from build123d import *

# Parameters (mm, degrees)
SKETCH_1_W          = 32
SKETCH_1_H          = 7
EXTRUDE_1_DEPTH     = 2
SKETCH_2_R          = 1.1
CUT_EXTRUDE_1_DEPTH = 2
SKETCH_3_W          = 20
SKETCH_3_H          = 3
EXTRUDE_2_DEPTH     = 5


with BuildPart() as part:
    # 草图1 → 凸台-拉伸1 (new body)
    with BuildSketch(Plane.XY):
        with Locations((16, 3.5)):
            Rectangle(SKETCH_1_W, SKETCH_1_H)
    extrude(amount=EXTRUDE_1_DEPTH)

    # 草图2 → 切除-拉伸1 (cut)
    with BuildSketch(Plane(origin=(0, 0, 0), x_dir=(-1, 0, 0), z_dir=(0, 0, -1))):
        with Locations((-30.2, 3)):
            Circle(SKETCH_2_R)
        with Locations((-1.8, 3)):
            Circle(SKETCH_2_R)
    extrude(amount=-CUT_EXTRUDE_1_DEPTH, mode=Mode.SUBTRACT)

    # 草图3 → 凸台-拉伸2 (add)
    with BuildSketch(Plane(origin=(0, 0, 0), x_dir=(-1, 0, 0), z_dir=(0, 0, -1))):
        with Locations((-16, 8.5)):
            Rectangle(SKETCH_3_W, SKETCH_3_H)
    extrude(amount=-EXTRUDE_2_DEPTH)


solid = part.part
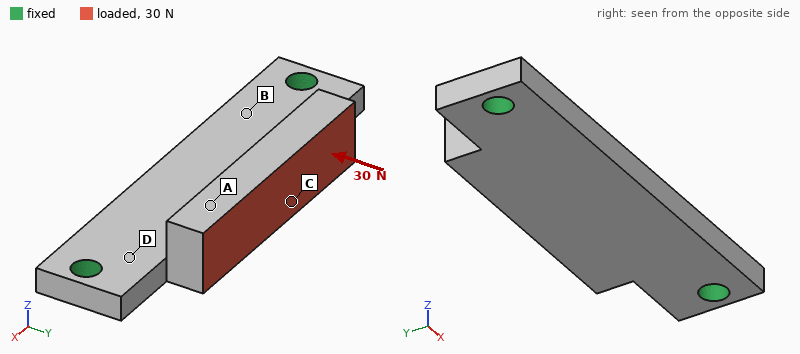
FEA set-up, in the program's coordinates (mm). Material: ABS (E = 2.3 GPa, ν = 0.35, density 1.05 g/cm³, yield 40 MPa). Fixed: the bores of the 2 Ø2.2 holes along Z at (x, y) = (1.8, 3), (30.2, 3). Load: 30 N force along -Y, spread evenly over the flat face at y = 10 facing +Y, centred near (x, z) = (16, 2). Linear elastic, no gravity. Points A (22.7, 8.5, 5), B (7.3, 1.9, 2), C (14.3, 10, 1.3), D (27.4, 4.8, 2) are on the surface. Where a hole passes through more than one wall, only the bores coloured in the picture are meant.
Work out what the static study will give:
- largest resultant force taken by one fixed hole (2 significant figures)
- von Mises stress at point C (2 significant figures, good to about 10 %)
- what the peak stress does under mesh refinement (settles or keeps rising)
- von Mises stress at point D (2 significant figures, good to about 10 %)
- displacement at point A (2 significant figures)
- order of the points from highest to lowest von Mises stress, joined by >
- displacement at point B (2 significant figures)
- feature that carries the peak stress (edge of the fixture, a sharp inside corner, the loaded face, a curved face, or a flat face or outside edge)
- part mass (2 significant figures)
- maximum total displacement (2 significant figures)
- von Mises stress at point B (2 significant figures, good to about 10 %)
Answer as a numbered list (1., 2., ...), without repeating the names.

1. 18 N
2. 2.3 MPa
3. keeps rising
4. 7.2 MPa
5. 0.094 mm
6. D > B > C > A
7. 0.022 mm
8. edge of the fixture
9. 0.77 g
10. 0.12 mm
11. 4.1 MPa
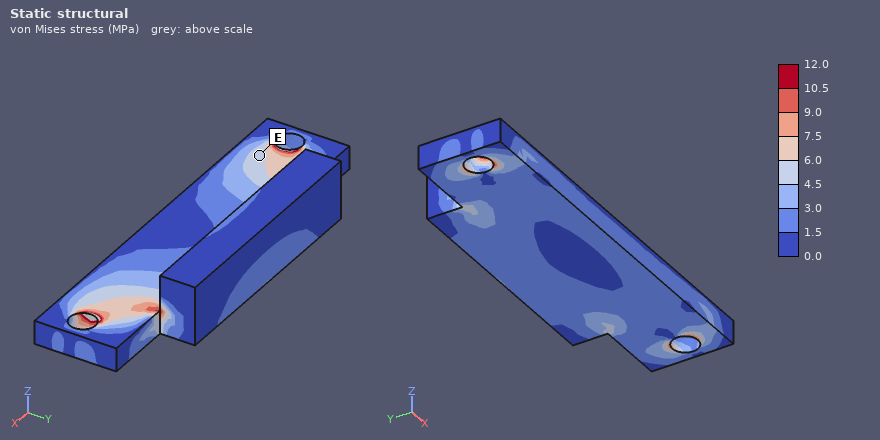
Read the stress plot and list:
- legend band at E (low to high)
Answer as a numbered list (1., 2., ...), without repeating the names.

1. 4.5 to 6.0 MPa
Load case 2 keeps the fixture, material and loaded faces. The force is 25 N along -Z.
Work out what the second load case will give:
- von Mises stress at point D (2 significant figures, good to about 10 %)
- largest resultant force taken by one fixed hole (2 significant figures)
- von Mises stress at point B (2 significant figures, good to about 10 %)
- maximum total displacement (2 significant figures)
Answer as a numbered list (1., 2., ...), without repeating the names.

1. 15 MPa
2. 13 N
3. 8.9 MPa
4. 0.34 mm
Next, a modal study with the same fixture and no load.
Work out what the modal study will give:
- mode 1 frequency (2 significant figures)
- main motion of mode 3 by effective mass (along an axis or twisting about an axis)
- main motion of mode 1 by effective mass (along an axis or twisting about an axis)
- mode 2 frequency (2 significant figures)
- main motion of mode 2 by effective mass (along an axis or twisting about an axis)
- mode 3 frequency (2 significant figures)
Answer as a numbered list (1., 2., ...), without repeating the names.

1. 2900 Hz
2. twisting about Y
3. along Z
4. 5200 Hz
5. along Z
6. 7700 Hz
